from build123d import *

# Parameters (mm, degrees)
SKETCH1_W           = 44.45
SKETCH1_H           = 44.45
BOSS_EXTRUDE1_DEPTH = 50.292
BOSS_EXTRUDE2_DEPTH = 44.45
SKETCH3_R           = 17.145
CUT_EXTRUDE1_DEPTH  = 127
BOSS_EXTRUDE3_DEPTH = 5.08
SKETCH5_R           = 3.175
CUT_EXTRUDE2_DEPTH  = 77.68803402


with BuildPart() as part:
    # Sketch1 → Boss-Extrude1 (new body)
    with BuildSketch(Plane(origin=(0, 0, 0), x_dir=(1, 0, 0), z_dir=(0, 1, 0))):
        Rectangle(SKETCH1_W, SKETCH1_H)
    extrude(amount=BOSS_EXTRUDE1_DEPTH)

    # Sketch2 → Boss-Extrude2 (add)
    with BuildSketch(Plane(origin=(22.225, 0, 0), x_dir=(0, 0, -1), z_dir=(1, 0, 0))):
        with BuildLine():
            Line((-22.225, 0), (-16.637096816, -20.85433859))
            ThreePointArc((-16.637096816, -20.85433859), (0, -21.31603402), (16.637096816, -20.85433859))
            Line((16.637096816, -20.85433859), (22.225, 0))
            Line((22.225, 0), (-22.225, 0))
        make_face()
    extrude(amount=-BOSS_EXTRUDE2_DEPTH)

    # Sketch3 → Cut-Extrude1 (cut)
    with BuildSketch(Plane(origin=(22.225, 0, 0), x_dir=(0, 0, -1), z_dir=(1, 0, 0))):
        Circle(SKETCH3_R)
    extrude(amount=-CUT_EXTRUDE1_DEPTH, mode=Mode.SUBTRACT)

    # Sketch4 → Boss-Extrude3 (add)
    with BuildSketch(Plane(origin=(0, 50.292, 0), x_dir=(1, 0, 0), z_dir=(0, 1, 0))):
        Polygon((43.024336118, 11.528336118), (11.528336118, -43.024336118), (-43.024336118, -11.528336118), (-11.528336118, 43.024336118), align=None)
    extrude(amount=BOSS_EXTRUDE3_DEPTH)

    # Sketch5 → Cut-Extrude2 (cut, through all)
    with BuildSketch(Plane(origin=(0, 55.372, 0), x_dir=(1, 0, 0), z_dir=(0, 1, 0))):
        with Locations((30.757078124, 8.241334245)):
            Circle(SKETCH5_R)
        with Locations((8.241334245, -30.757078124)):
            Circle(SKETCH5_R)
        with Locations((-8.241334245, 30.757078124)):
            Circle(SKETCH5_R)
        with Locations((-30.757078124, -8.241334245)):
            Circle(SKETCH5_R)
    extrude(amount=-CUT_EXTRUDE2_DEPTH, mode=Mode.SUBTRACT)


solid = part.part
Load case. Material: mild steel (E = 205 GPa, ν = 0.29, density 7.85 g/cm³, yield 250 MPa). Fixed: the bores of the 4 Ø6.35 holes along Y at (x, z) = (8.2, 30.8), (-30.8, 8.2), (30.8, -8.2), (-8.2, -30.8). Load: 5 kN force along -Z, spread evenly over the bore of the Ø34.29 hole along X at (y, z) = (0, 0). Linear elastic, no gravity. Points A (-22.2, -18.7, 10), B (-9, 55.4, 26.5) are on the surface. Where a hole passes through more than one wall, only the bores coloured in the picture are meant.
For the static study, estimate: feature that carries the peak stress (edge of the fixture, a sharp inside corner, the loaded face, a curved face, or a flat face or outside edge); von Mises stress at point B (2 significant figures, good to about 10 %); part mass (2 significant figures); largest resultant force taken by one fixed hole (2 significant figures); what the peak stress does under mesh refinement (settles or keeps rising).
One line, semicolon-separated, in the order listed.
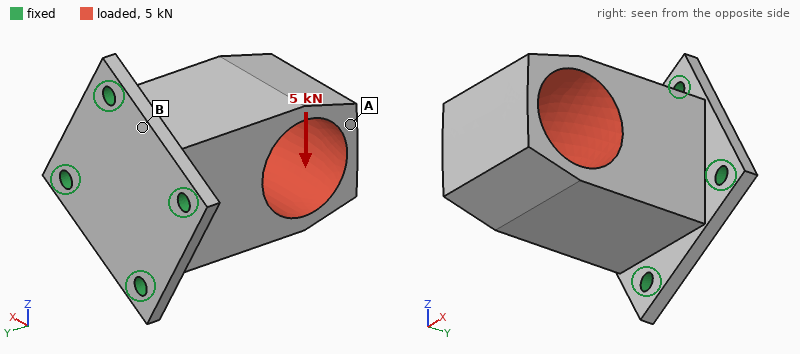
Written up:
edge of the fixture; 50 MPa; 900 g; 4.9 kN; keeps rising
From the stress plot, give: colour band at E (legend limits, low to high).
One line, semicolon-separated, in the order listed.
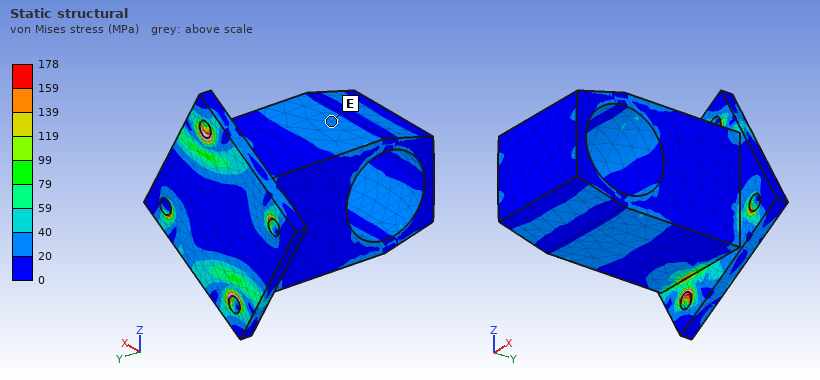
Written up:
20 to 40 MPa
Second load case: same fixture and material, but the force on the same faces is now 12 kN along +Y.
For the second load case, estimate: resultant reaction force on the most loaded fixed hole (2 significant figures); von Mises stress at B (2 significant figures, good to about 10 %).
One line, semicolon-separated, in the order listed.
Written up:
3.2 kN; 28 MPa
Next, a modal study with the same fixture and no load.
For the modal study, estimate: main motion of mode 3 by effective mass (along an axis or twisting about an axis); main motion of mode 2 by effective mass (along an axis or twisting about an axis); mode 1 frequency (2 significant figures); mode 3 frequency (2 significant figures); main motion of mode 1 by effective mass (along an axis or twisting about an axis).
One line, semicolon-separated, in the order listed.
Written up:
along Y; along X; 2900 Hz; 6000 Hz; along Z
